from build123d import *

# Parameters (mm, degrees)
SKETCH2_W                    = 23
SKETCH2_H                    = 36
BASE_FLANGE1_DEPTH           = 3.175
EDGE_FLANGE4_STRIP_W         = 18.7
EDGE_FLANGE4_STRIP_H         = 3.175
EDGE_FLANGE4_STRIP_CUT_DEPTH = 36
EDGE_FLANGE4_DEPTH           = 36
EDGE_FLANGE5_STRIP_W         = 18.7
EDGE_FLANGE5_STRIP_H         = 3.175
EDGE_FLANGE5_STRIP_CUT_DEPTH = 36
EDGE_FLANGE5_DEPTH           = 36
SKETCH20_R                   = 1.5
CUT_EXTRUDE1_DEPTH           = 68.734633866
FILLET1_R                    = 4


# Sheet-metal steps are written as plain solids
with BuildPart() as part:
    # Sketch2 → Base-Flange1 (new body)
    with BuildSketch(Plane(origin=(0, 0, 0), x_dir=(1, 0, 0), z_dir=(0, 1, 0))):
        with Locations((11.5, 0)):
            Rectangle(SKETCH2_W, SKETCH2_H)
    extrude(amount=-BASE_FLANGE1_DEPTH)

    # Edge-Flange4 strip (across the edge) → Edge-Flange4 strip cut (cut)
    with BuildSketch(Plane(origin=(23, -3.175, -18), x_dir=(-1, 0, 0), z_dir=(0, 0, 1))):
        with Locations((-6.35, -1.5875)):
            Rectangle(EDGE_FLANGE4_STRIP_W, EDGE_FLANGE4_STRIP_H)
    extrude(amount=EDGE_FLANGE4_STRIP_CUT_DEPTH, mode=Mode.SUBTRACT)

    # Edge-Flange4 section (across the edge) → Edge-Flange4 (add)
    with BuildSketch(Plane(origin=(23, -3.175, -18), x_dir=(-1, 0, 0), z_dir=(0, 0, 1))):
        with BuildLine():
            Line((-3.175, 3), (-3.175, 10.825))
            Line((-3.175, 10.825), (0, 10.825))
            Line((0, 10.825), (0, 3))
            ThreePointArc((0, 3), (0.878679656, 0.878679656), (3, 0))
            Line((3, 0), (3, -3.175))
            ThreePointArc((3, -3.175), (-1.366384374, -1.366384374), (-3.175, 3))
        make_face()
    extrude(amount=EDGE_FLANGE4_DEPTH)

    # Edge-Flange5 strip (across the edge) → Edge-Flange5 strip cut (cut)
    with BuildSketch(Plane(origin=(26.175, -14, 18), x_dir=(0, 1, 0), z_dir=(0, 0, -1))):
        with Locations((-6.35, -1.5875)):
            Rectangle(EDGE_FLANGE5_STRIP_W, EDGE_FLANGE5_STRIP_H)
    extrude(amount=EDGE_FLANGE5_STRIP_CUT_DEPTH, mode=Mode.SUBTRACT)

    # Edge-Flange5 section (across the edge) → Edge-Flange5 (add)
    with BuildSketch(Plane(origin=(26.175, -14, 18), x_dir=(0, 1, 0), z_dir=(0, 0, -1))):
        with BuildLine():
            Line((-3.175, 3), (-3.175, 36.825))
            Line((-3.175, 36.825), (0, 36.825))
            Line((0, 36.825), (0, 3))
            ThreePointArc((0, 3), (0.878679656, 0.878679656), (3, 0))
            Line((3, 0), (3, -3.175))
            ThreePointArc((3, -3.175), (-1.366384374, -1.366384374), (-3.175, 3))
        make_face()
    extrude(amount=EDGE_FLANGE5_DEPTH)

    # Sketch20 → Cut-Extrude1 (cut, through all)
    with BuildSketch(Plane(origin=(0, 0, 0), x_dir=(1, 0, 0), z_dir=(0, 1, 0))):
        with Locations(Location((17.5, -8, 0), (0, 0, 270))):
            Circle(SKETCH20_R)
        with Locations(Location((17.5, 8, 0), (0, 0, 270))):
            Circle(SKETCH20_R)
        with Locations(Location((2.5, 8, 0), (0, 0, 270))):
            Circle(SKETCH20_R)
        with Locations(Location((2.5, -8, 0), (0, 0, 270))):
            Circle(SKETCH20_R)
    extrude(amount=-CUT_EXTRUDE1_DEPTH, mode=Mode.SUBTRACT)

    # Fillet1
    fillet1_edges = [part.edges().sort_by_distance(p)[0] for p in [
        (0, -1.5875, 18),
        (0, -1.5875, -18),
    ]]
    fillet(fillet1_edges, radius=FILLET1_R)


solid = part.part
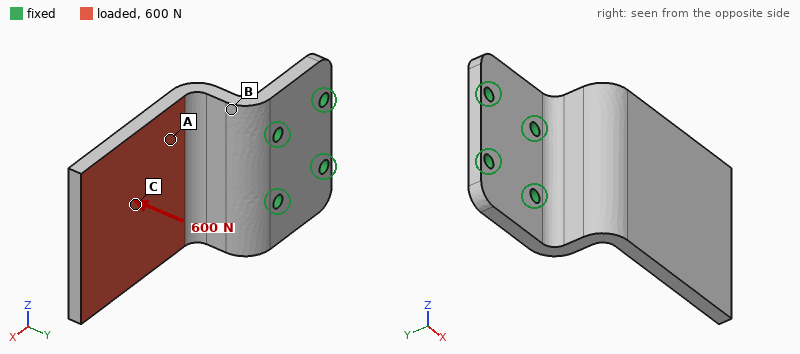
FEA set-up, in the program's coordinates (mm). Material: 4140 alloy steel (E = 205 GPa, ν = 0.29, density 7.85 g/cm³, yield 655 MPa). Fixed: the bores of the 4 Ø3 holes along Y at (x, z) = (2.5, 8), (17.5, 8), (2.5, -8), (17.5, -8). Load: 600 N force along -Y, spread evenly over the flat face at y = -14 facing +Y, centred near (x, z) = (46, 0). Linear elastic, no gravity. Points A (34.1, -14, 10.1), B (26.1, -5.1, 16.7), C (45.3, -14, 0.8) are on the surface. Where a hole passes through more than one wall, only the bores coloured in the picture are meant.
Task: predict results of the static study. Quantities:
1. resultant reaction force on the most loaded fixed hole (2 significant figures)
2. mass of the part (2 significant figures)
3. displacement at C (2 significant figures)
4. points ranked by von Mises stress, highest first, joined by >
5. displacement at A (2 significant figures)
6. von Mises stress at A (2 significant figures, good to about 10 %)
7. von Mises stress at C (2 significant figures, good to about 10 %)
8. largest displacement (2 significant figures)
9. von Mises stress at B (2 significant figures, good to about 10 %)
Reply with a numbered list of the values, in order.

1. 480 N
2. 65 g
3. 0.37 mm
4. B > A > C
5. 0.18 mm
6. 110 MPa
7. 44 MPa
8. 0.72 mm
9. 180 MPa
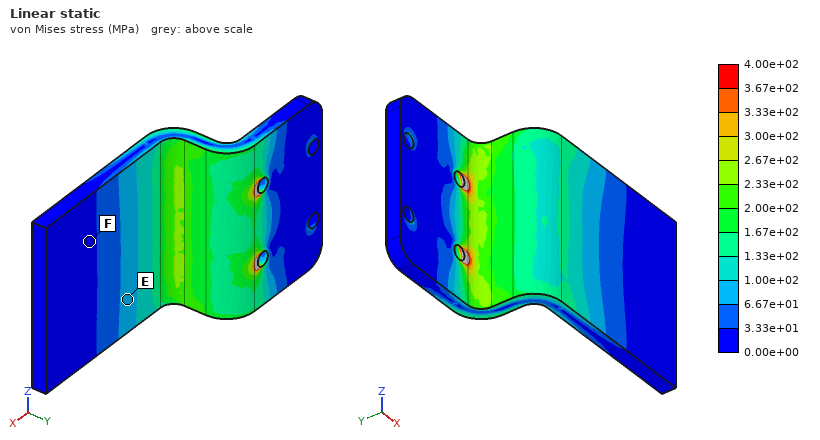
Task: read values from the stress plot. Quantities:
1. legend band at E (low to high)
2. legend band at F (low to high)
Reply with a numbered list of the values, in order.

1. 6.67e+01 to 1.00e+02 MPa
2. 0.00e+00 to 3.33e+01 MPa
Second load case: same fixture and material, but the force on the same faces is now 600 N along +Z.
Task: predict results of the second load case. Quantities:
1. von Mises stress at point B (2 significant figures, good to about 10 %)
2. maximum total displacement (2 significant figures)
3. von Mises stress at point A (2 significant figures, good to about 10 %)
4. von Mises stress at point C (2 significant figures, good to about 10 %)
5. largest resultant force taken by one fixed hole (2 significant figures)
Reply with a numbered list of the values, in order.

1. 76 MPa
2. 0.12 mm
3. 55 MPa
4. 22 MPa
5. 790 N
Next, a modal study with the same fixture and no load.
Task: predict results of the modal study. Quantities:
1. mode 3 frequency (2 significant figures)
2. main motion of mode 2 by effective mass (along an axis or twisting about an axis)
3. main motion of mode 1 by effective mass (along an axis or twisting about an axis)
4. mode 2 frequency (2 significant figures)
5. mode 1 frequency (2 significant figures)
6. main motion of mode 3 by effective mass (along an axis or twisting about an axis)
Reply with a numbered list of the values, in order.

1. 4200 Hz
2. along Z
3. along Y
4. 2400 Hz
5. 980 Hz
6. along X
